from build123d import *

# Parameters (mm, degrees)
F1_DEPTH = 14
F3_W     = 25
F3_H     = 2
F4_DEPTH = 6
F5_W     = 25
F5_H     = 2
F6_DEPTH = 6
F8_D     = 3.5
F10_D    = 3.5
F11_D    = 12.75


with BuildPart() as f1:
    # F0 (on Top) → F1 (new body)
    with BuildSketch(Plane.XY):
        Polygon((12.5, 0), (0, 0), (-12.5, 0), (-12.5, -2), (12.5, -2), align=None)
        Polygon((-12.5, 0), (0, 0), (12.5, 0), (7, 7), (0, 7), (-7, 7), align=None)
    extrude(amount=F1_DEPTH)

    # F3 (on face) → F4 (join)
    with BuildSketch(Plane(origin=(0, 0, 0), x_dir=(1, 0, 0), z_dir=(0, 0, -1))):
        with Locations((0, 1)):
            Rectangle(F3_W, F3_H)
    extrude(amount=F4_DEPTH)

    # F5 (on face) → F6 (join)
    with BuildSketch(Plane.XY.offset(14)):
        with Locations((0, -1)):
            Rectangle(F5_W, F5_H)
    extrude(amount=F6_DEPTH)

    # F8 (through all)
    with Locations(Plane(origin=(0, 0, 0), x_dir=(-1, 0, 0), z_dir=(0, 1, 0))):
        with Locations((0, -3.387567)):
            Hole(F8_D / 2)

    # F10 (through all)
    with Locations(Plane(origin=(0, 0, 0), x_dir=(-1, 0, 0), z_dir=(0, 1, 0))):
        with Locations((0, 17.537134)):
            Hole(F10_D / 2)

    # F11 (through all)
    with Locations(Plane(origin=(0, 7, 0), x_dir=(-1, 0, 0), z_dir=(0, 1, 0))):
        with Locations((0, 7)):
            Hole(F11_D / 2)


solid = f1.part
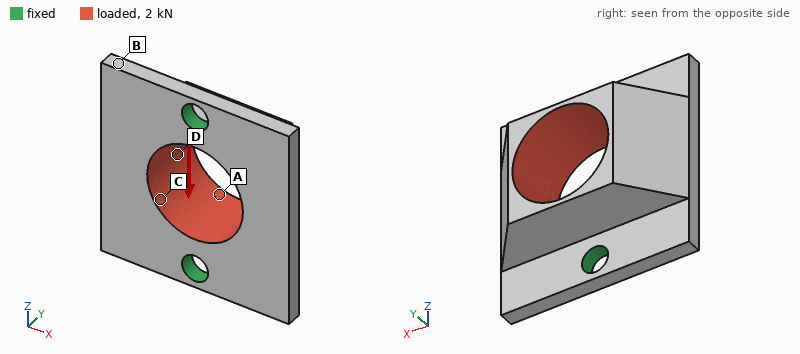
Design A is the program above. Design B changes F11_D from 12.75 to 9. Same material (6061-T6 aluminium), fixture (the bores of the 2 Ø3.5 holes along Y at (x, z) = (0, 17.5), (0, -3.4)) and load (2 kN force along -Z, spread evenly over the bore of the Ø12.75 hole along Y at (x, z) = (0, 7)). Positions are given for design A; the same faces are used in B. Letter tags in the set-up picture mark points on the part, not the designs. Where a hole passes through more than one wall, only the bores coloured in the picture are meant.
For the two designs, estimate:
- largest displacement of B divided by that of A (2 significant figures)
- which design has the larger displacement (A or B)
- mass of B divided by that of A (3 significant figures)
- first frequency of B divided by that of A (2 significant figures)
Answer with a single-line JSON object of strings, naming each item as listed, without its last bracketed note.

{"largest displacement of B divided by that of A": "0.50", "which design has the larger displacement": "A", "mass of B divided by that of A": "1.28", "first frequency of B divided by that of A": "0.98"}
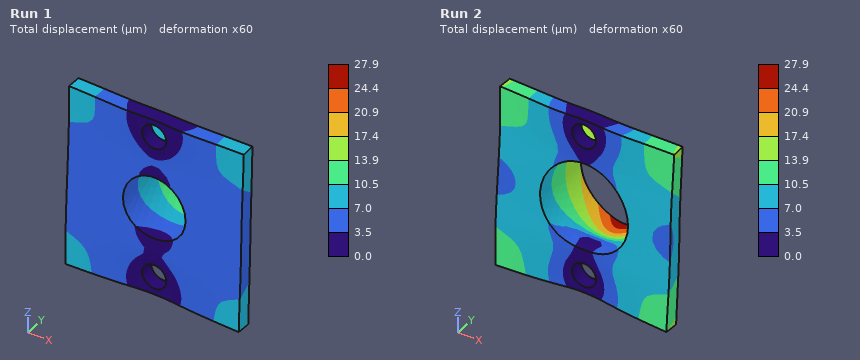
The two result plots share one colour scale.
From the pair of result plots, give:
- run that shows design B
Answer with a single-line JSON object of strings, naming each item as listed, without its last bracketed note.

{"run that shows design B": "Run 1"}
